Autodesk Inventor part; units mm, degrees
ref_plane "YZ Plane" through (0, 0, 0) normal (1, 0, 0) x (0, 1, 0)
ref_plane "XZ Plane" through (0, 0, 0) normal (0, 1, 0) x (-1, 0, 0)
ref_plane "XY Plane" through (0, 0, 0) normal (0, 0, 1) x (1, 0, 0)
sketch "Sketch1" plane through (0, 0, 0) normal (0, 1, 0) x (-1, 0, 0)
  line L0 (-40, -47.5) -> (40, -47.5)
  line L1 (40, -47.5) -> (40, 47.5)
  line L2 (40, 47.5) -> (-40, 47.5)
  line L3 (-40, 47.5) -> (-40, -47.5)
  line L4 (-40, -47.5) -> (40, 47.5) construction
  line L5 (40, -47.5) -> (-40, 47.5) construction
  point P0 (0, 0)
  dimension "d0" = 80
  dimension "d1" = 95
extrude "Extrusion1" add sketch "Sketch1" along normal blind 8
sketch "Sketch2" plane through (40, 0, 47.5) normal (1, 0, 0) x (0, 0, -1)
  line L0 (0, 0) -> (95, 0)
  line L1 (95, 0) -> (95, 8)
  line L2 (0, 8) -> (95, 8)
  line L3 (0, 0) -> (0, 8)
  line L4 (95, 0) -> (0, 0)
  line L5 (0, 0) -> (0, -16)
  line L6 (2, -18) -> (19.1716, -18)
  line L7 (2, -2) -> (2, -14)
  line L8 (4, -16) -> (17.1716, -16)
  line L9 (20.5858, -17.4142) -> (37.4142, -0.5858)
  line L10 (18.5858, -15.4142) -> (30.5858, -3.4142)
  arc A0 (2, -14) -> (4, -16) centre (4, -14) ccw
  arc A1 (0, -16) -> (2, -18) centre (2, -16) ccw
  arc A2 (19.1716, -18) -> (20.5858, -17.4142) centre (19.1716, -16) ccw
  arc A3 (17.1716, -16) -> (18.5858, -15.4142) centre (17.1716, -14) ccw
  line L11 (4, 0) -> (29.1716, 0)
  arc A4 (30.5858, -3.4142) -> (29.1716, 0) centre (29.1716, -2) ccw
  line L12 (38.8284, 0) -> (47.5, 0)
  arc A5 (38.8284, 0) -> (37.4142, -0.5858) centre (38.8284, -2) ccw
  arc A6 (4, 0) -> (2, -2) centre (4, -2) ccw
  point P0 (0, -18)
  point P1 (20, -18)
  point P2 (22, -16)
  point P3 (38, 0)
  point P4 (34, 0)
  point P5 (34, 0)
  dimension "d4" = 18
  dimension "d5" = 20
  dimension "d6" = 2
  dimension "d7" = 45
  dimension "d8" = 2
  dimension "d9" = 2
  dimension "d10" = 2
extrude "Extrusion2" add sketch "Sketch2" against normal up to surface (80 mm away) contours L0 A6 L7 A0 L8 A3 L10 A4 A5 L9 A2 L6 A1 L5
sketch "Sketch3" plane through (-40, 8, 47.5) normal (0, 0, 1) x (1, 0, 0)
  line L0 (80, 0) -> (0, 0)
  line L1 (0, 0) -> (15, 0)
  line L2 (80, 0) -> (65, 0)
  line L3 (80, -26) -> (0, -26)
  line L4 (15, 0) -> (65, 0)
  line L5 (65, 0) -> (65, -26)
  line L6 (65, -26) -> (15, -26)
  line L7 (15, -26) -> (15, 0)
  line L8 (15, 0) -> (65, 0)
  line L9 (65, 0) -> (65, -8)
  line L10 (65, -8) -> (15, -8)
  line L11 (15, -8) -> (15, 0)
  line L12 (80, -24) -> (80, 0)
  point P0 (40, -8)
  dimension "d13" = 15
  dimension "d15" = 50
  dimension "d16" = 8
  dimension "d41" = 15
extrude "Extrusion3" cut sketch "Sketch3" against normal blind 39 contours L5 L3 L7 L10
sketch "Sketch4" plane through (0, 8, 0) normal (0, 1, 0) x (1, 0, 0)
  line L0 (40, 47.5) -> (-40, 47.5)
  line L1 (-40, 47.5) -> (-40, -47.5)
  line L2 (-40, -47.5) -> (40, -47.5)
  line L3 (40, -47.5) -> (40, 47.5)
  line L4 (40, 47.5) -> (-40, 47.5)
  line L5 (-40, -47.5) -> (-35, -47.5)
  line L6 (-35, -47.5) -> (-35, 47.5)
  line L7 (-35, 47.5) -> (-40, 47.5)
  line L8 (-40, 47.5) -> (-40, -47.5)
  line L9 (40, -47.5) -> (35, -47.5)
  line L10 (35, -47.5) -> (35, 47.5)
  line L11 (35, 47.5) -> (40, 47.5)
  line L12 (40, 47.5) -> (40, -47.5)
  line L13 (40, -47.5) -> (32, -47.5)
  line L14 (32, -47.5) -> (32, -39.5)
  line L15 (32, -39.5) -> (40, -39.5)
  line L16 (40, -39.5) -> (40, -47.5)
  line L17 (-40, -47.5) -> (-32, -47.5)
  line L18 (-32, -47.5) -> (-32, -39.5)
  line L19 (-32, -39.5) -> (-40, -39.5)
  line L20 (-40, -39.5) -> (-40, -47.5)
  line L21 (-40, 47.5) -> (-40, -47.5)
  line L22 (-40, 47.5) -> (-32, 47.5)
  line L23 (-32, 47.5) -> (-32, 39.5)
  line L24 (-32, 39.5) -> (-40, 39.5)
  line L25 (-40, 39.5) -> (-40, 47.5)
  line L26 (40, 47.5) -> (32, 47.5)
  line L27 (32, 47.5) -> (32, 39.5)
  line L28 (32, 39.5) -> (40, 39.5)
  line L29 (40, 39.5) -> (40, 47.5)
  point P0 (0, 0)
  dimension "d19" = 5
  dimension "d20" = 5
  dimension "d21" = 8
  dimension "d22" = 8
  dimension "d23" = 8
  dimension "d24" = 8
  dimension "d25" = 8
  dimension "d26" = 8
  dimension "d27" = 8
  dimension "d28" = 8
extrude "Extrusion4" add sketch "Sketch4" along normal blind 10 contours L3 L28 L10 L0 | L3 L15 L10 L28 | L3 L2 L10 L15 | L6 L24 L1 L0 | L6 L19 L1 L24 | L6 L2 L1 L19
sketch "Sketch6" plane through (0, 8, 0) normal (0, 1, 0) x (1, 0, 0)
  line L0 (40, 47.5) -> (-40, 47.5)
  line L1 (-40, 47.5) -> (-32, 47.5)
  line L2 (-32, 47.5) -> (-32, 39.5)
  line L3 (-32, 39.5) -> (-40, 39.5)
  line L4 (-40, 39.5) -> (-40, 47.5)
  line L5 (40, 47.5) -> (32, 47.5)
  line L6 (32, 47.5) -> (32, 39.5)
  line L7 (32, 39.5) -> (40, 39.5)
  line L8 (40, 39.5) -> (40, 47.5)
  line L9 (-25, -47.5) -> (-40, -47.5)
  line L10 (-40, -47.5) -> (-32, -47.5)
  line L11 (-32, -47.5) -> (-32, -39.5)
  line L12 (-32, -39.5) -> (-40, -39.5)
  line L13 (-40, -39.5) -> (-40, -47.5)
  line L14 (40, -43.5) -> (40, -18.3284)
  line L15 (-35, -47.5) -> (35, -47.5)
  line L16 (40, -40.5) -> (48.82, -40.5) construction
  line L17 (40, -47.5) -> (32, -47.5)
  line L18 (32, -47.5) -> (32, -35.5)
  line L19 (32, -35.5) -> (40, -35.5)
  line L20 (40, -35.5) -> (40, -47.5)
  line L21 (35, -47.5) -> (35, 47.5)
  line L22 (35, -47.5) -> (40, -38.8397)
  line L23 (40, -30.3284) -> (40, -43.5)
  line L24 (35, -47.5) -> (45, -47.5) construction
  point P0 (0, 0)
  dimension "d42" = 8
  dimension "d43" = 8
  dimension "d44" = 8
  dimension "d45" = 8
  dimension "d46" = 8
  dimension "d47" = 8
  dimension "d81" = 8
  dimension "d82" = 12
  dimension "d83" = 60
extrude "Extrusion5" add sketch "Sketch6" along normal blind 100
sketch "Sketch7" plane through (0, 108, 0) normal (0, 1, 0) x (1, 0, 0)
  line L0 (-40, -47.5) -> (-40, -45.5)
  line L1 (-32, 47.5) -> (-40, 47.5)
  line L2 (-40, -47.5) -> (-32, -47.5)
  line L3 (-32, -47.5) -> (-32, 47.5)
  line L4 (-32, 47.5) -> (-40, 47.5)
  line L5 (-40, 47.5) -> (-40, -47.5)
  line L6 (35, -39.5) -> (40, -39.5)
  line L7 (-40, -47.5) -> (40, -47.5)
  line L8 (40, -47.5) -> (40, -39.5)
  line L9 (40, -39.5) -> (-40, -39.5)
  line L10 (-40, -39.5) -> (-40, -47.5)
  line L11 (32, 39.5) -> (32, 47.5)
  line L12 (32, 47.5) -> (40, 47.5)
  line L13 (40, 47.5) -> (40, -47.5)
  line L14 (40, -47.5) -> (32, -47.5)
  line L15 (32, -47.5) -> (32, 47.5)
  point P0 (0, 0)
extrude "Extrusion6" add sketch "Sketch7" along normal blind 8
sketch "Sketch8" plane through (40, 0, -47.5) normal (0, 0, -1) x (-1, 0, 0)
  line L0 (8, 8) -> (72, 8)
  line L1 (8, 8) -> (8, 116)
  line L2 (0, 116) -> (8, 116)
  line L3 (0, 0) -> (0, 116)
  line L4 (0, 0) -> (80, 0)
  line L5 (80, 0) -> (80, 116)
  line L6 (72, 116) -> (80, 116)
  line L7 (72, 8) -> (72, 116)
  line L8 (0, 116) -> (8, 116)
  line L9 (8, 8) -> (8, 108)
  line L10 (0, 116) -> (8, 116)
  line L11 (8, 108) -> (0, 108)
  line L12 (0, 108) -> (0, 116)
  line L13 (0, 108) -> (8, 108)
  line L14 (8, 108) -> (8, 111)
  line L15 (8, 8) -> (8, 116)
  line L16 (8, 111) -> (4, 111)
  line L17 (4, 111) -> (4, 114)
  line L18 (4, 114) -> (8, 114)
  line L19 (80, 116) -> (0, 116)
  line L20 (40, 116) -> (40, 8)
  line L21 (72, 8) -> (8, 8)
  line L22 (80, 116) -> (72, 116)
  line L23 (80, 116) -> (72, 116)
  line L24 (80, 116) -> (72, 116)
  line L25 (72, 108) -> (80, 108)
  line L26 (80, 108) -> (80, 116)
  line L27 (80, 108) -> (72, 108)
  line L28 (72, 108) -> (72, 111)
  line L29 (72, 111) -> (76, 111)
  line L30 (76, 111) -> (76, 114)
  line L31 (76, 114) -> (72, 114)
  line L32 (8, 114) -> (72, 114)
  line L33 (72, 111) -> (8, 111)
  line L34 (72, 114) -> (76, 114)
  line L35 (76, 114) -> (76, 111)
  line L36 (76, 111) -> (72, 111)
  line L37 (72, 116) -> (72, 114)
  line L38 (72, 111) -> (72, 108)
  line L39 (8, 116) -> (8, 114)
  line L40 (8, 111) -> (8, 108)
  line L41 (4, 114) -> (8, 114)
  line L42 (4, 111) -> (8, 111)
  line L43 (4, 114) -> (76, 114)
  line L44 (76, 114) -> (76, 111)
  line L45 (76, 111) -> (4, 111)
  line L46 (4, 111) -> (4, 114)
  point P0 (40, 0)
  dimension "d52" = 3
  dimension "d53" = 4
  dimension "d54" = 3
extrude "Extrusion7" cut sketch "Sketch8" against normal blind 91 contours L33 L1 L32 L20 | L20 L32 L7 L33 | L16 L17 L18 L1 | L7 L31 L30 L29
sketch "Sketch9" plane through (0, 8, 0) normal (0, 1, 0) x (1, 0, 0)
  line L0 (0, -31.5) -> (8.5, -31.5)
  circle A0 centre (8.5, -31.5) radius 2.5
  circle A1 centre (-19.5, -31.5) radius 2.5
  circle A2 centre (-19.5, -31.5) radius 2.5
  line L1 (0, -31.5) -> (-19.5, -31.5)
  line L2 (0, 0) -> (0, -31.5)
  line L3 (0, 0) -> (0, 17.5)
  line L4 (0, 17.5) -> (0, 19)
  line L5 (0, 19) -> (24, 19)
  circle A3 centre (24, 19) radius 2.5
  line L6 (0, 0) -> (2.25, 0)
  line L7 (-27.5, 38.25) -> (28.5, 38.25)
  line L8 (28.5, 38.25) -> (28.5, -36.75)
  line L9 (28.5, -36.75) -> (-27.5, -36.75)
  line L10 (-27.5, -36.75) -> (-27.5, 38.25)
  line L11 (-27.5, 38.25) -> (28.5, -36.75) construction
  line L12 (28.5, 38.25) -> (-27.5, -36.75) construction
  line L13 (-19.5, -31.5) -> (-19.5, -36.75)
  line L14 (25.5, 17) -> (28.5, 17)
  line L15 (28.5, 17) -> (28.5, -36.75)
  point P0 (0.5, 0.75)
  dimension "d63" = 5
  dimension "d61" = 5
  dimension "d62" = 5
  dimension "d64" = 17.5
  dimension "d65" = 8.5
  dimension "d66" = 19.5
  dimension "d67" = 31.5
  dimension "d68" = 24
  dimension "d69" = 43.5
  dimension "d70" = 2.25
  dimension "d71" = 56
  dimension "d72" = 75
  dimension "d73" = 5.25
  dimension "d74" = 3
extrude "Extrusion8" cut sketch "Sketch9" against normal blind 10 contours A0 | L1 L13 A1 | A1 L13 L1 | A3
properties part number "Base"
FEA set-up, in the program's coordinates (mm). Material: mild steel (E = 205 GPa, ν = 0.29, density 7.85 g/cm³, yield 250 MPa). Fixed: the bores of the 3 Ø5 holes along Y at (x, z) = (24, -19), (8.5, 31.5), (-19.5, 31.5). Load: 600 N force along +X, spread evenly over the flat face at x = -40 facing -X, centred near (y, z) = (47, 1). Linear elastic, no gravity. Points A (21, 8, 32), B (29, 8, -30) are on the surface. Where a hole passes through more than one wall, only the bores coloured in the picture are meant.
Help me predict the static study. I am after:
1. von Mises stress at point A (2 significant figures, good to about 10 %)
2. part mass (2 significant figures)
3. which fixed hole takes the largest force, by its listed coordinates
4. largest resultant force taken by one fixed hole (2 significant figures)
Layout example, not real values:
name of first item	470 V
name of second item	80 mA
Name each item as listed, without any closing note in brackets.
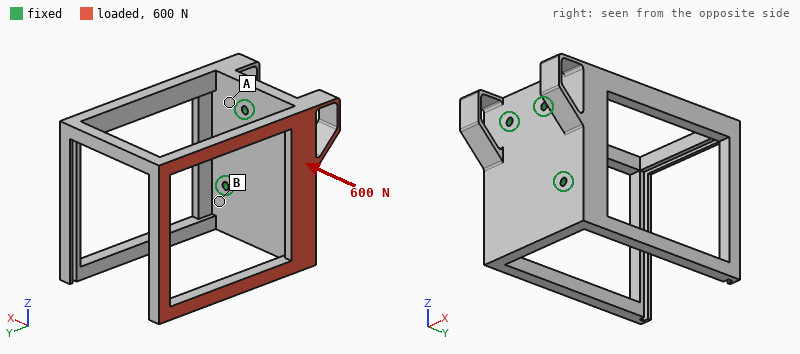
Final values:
von Mises stress at point A	12 MPa
part mass	900 g
which fixed hole takes the largest force, by its listed coordinates	(-19.5, 31.5)
largest resultant force taken by one fixed hole	490 N
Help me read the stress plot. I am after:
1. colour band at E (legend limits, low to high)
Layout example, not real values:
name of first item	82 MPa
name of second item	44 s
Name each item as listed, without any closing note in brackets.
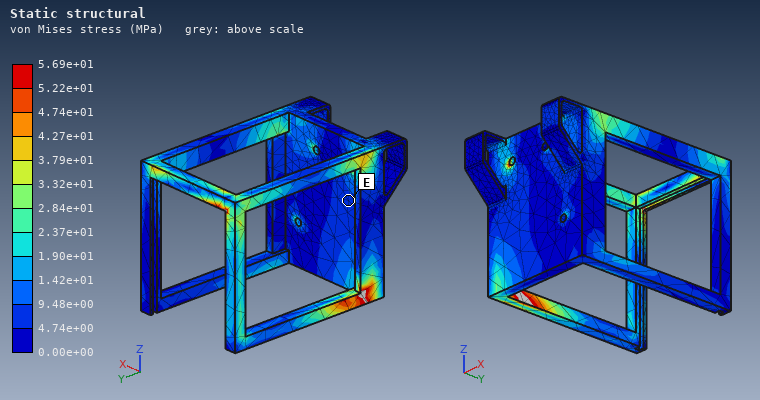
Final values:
colour band at E	4.74e+00 to 9.48e+00 MPa
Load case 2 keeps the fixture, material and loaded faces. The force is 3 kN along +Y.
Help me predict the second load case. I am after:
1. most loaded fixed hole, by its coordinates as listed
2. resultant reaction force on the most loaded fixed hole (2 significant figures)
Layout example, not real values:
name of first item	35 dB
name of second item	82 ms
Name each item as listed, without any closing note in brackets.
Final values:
most loaded fixed hole, by its coordinates as listed	(-19.5, 31.5)
resultant reaction force on the most loaded fixed hole	3.4 kN
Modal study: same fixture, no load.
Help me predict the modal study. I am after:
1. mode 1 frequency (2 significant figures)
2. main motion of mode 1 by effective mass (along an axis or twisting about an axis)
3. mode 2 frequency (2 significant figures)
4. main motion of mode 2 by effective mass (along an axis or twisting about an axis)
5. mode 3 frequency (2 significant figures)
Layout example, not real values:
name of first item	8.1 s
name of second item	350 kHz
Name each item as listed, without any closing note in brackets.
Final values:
mode 1 frequency	450 Hz
main motion of mode 1 by effective mass	along X
mode 2 frequency	580 Hz
main motion of mode 2 by effective mass	along Z
mode 3 frequency	650 Hz
